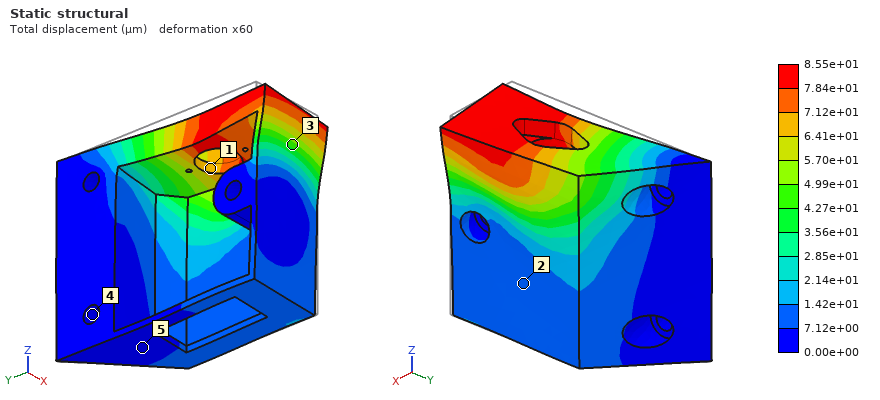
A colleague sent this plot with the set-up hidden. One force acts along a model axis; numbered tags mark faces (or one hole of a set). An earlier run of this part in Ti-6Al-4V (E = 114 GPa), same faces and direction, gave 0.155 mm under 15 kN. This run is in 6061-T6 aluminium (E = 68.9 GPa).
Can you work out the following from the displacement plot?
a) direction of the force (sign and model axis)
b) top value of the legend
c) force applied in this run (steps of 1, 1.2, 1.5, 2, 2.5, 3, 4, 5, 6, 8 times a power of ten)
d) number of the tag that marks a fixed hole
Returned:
+X
8.55e+01 µm
5 kN
4
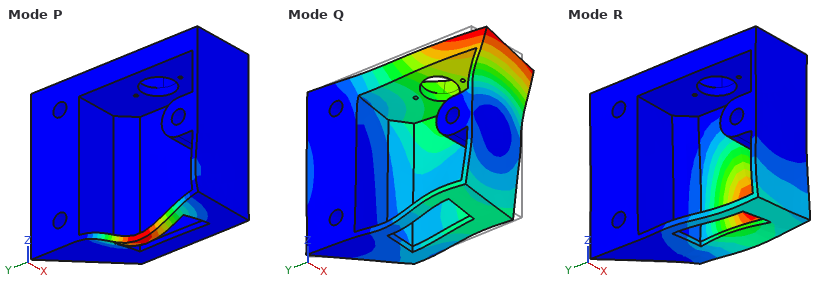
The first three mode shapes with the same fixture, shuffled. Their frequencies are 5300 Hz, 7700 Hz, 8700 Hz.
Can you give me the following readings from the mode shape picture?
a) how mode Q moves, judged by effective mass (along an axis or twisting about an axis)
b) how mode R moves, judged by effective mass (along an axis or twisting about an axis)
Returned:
along X
along X
